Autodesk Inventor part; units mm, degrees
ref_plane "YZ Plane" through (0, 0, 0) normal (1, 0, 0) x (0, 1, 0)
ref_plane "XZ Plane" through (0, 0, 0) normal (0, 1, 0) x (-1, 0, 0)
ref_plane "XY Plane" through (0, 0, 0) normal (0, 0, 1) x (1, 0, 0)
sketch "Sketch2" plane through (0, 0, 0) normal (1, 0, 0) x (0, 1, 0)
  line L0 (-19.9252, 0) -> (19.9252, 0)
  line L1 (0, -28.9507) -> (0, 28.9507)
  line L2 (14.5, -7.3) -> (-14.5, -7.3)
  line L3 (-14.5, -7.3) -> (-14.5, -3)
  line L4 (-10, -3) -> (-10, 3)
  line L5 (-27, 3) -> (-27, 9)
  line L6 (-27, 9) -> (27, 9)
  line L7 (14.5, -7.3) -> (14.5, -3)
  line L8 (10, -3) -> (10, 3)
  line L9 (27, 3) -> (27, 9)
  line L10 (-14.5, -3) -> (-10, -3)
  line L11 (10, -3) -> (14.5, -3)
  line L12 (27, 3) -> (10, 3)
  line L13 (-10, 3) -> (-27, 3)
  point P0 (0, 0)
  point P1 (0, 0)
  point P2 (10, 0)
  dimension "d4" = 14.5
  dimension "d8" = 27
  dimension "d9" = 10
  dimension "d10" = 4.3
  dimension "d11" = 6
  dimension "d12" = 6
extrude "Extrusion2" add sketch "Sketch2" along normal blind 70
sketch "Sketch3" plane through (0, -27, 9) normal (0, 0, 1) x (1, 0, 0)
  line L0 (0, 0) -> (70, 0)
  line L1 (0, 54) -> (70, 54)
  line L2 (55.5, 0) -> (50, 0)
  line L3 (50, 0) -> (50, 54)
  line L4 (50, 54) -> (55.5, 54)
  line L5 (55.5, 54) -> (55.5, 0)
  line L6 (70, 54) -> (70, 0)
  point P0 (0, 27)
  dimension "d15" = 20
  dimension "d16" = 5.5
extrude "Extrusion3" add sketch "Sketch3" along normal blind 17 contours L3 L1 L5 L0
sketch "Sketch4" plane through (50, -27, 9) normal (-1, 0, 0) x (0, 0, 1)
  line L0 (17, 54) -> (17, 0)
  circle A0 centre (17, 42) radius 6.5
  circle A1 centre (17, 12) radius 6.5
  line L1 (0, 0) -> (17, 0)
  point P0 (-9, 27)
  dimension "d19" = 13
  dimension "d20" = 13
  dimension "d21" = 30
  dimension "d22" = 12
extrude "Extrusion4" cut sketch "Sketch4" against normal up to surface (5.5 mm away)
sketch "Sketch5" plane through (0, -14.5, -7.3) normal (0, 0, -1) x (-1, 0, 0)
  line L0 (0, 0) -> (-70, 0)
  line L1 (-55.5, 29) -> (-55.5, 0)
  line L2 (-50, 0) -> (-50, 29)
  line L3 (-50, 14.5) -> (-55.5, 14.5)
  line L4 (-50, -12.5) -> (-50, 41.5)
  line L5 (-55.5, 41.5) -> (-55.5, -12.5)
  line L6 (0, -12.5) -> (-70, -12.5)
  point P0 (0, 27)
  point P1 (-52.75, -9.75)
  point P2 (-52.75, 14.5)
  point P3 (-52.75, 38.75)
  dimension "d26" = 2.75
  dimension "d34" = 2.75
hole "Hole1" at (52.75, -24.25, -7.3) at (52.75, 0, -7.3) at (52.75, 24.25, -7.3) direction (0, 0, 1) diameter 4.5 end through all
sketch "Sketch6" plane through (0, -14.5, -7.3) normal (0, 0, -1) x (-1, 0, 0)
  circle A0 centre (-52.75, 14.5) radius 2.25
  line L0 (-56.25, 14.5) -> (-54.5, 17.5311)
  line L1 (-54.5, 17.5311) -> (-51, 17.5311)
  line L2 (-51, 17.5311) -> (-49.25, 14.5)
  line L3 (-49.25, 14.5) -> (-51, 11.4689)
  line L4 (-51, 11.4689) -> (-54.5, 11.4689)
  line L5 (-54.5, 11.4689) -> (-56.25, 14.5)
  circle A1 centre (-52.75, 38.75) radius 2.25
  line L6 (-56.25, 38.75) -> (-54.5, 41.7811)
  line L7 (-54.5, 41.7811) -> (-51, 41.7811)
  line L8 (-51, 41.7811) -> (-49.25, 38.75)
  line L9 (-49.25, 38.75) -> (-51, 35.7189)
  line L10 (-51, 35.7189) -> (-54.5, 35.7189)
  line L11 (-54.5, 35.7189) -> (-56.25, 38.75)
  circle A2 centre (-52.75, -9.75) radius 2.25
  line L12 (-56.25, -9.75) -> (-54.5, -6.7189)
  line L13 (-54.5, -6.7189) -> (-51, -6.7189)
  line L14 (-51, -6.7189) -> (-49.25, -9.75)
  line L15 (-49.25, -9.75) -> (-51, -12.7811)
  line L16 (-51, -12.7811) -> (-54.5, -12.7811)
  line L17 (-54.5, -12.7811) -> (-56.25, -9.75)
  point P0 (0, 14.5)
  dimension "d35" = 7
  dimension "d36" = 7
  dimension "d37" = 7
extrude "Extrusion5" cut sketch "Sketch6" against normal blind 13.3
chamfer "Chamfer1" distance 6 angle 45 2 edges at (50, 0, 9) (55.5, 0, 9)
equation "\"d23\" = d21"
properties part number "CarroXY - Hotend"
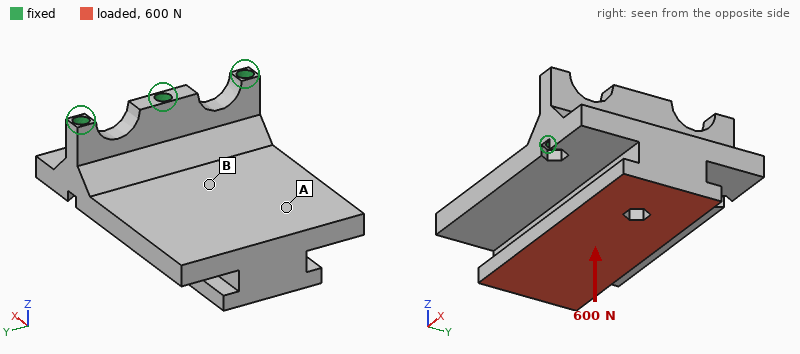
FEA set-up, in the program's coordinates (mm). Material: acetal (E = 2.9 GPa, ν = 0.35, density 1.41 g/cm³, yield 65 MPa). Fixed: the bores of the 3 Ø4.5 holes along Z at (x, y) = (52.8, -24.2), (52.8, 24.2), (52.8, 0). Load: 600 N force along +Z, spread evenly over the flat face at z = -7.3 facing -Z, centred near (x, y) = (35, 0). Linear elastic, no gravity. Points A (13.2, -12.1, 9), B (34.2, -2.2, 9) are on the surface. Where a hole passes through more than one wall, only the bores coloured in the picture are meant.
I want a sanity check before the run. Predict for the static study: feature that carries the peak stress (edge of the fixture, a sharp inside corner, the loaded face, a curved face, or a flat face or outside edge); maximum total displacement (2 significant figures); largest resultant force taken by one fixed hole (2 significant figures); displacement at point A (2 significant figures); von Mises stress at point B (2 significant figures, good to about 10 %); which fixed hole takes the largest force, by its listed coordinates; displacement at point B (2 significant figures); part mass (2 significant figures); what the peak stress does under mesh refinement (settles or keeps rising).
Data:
edge of the fixture
0.63 mm
440 N
0.43 mm
3.8 MPa
(52.8, 0)
0.17 mm
63 g
keeps rising
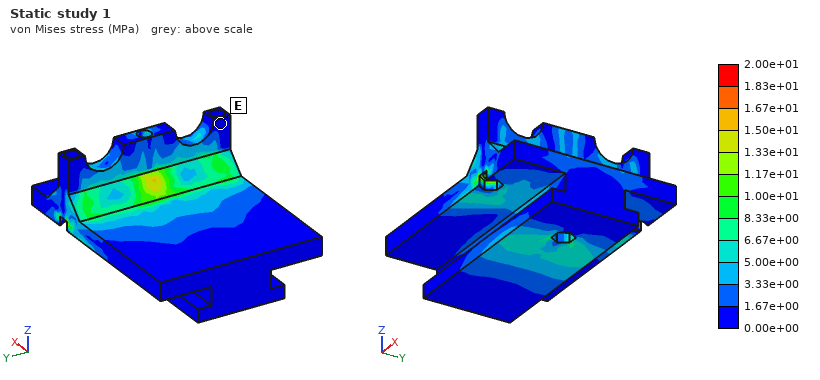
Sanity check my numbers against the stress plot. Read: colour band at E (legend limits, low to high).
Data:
0.00e+00 to 1.67e+00 MPa
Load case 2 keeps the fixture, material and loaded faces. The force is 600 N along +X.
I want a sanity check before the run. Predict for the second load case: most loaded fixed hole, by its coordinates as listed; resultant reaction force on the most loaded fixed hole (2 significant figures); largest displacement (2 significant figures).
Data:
(52.8, 0)
370 N
0.50 mm
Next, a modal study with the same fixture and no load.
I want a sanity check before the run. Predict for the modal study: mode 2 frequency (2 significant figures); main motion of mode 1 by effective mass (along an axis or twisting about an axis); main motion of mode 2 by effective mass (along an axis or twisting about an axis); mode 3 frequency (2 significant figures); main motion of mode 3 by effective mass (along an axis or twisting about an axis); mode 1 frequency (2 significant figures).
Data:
1900 Hz
along Z
twisting about X
2300 Hz
along Y
790 Hz
